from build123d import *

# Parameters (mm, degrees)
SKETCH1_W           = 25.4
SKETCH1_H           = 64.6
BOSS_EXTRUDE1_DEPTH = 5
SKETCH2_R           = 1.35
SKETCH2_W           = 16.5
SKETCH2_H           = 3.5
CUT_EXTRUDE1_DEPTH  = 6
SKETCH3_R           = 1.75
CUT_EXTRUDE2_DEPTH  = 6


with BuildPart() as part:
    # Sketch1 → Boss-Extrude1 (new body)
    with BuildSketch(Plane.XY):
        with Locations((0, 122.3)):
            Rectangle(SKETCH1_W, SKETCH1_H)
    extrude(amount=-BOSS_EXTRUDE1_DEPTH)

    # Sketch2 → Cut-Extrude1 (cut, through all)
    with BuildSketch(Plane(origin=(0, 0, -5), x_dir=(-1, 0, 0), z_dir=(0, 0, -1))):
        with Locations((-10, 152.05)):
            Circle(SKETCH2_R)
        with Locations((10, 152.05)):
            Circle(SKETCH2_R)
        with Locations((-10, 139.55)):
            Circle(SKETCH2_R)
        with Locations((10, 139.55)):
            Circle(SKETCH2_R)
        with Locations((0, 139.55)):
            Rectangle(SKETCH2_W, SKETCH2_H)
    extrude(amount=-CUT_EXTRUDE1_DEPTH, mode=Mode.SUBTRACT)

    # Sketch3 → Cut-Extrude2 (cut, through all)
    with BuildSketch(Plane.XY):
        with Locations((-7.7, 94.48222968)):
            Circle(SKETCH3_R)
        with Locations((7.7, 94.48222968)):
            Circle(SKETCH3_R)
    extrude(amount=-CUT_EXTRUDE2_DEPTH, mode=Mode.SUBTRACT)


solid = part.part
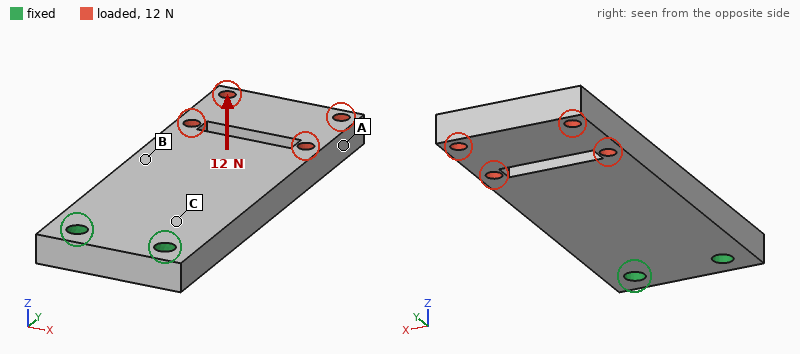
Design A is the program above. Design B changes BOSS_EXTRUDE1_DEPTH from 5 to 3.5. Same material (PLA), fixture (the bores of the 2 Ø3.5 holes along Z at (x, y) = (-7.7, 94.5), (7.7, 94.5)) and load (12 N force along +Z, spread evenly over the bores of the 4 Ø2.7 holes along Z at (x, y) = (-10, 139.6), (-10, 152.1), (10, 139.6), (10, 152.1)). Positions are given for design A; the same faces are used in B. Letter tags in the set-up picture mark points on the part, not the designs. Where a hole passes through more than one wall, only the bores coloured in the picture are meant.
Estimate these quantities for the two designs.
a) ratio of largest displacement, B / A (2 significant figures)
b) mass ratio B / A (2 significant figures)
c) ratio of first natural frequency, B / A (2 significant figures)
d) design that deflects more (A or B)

2.8
0.70
0.71
B
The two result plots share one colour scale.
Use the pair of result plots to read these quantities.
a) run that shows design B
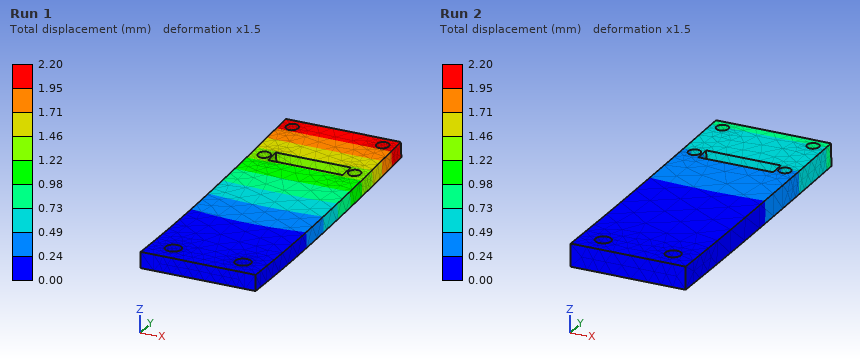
Run 1
